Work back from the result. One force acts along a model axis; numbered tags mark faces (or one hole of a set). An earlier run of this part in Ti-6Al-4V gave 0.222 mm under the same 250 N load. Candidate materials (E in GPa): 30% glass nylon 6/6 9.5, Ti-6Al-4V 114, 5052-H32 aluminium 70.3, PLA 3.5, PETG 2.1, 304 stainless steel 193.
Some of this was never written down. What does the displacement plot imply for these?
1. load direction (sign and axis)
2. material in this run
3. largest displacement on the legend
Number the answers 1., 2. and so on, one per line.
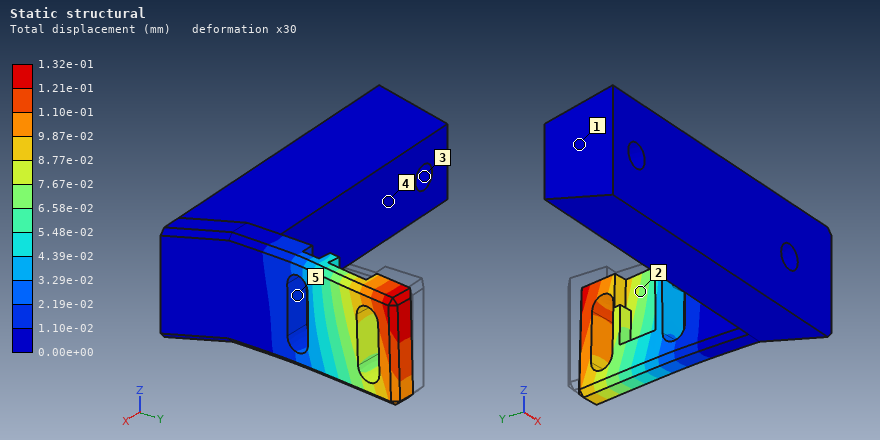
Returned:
1. +X
2. 304 stainless steel
3. 1.32e-01 mm
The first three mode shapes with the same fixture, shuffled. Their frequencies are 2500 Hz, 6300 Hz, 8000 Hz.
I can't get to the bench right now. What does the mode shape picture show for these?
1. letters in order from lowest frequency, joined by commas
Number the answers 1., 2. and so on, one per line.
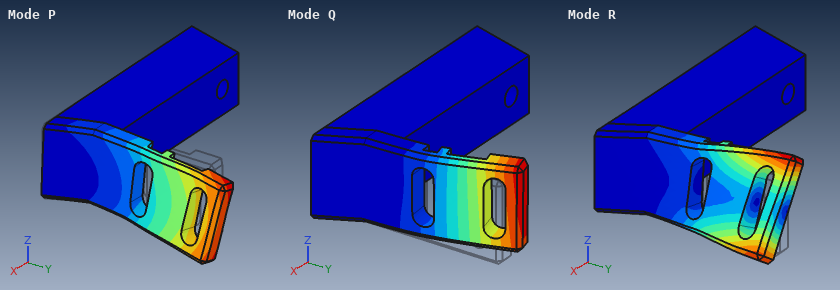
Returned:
1. Q, P, R
